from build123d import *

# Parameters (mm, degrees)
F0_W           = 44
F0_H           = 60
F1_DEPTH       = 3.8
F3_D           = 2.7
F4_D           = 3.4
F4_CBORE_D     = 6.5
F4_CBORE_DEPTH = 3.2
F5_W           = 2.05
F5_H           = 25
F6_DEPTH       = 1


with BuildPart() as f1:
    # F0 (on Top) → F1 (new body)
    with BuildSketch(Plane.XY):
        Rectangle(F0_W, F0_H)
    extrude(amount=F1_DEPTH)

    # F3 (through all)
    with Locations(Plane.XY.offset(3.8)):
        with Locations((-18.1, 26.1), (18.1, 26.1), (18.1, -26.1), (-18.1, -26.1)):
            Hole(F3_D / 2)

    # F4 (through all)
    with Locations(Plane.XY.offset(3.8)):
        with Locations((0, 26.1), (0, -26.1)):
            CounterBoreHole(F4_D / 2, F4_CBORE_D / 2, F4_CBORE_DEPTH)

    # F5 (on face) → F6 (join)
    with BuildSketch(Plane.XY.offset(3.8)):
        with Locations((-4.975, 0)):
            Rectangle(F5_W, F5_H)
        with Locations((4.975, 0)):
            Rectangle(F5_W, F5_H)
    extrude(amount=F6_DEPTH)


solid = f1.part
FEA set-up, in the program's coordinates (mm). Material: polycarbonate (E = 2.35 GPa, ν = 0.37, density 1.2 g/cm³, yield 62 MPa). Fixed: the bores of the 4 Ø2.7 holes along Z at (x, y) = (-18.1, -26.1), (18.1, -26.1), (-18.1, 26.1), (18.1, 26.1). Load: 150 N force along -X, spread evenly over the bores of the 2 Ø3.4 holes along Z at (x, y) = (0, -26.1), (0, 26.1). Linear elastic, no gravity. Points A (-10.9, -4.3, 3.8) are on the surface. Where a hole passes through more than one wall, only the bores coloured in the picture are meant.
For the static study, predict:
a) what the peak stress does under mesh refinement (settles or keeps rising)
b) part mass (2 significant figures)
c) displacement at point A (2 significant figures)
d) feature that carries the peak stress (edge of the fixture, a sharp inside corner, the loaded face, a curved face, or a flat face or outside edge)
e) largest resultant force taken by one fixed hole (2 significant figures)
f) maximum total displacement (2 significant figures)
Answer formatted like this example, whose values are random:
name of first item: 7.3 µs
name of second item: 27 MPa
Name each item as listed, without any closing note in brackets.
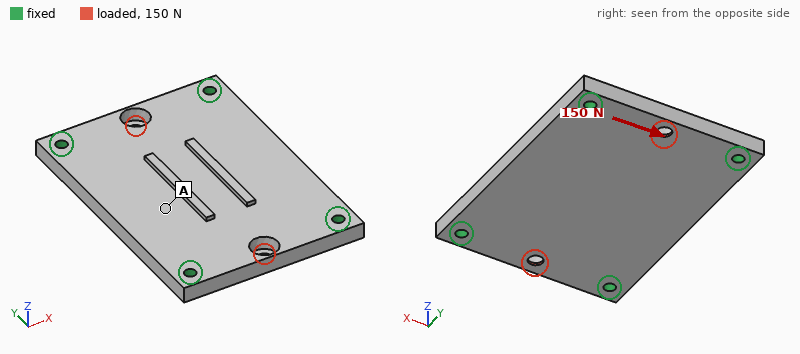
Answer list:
what the peak stress does under mesh refinement: keeps rising
part mass: 12 g
displacement at point A: 4.1 µm
feature that carries the peak stress: a sharp inside corner
largest resultant force taken by one fixed hole: 38 N
maximum total displacement: 25 µm
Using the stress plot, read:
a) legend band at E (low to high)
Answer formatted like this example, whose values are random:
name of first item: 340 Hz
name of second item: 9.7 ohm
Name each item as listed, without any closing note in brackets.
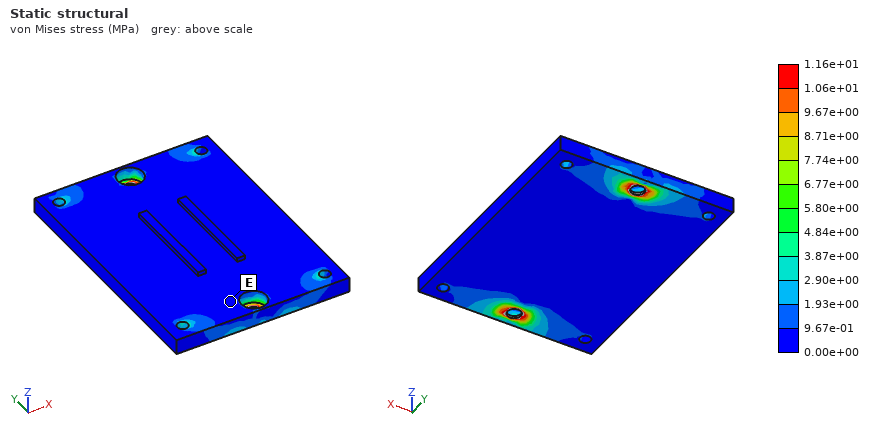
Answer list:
legend band at E: 0.00e+00 to 9.67e-01 MPa
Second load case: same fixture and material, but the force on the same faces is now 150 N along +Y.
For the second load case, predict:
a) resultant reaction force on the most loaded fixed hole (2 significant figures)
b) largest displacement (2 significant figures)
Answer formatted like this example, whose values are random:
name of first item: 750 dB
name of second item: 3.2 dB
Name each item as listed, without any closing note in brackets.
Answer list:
resultant reaction force on the most loaded fixed hole: 40 N
largest displacement: 56 µm
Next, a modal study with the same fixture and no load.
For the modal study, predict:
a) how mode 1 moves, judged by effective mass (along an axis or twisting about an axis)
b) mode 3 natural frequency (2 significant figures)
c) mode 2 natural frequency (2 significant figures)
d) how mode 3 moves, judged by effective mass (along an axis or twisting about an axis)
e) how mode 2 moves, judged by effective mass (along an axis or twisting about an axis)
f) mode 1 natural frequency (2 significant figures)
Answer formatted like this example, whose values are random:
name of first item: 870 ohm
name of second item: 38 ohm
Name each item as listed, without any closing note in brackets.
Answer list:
how mode 1 moves, judged by effective mass: along Z
mode 3 natural frequency: 3600 Hz
mode 2 natural frequency: 2400 Hz
how mode 3 moves, judged by effective mass: twisting about X
how mode 2 moves, judged by effective mass: twisting about Y
mode 1 natural frequency: 1600 Hz
